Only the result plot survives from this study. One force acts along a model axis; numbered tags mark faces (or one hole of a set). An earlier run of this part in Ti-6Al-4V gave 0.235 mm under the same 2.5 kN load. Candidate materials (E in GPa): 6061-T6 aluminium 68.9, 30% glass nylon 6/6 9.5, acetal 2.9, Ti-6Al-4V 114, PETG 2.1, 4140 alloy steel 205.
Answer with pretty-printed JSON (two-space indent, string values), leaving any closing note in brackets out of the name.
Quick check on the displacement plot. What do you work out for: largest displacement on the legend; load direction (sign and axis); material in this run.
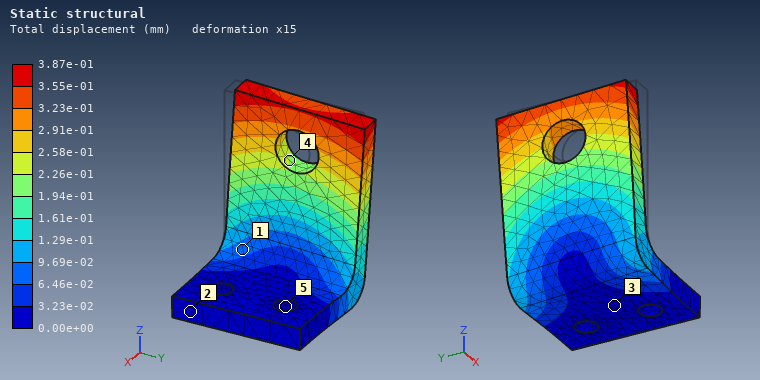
{
  "largest displacement on the legend": "3.87e-01 mm",
  "load direction": "+Y",
  "material in this run": "6061-T6 aluminium"
}
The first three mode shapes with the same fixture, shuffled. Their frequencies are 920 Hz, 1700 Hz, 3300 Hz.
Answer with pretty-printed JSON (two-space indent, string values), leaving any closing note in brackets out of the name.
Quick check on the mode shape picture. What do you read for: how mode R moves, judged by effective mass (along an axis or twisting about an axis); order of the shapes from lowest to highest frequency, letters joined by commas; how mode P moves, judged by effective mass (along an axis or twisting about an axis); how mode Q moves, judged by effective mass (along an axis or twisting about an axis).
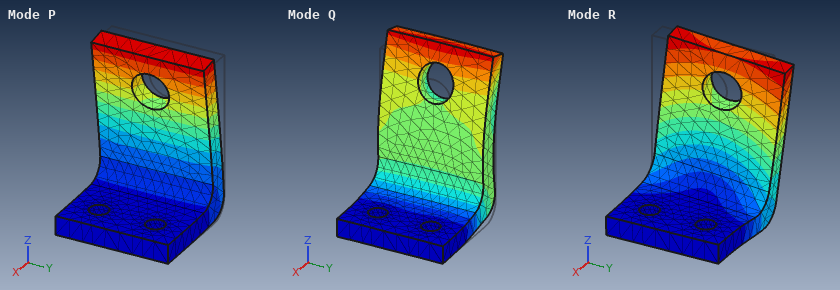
{
  "how mode R moves, judged by effective mass": "along Y",
  "order of the shapes from lowest to highest frequency, letters joined by commas": "P, R, Q",
  "how mode P moves, judged by effective mass": "along X",
  "how mode Q moves, judged by effective mass": "along Z"
}
